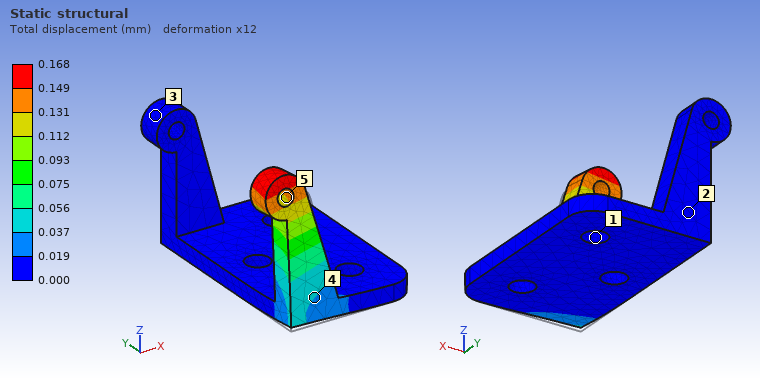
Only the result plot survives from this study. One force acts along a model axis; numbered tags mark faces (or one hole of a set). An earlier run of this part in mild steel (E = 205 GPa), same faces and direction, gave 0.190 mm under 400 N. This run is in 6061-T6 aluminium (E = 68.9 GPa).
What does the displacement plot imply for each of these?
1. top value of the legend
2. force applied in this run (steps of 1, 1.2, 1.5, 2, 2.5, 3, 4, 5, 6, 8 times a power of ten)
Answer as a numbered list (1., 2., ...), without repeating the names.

1. 0.168 mm
2. 120 N
